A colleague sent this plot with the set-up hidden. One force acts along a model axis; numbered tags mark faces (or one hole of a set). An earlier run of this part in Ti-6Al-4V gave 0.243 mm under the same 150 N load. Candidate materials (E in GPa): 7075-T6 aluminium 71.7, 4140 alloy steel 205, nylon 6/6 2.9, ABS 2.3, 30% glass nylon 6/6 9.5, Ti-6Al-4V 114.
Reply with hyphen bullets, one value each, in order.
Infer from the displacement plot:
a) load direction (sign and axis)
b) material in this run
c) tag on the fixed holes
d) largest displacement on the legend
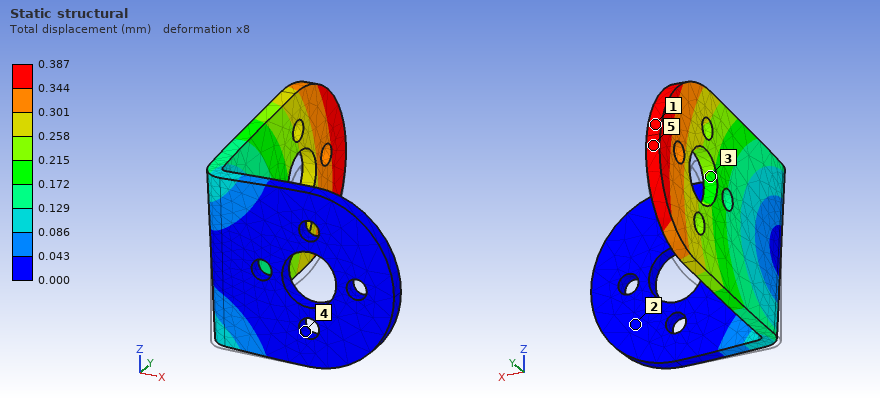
- +Z
- 7075-T6 aluminium
- 4
- 0.387 mm
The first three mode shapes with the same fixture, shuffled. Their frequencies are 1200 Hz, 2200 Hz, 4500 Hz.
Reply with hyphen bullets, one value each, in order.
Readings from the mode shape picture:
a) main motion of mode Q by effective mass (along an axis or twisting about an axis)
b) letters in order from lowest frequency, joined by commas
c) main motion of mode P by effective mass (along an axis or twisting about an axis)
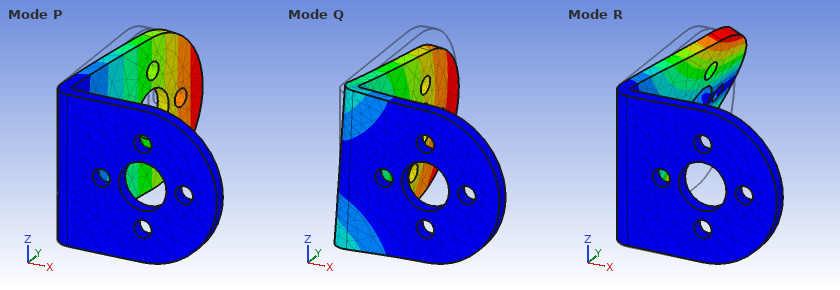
- along Z
- P, Q, R
- along X
